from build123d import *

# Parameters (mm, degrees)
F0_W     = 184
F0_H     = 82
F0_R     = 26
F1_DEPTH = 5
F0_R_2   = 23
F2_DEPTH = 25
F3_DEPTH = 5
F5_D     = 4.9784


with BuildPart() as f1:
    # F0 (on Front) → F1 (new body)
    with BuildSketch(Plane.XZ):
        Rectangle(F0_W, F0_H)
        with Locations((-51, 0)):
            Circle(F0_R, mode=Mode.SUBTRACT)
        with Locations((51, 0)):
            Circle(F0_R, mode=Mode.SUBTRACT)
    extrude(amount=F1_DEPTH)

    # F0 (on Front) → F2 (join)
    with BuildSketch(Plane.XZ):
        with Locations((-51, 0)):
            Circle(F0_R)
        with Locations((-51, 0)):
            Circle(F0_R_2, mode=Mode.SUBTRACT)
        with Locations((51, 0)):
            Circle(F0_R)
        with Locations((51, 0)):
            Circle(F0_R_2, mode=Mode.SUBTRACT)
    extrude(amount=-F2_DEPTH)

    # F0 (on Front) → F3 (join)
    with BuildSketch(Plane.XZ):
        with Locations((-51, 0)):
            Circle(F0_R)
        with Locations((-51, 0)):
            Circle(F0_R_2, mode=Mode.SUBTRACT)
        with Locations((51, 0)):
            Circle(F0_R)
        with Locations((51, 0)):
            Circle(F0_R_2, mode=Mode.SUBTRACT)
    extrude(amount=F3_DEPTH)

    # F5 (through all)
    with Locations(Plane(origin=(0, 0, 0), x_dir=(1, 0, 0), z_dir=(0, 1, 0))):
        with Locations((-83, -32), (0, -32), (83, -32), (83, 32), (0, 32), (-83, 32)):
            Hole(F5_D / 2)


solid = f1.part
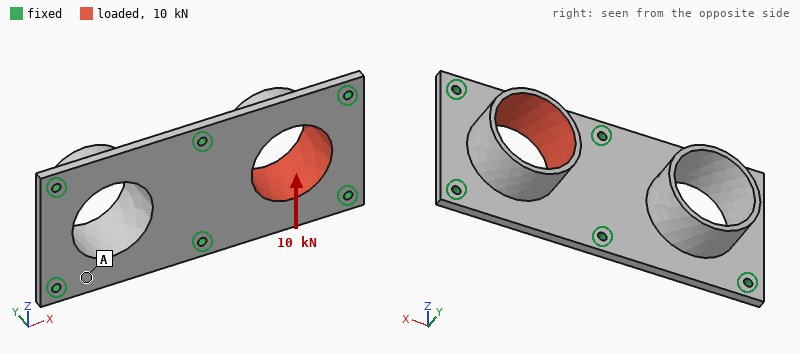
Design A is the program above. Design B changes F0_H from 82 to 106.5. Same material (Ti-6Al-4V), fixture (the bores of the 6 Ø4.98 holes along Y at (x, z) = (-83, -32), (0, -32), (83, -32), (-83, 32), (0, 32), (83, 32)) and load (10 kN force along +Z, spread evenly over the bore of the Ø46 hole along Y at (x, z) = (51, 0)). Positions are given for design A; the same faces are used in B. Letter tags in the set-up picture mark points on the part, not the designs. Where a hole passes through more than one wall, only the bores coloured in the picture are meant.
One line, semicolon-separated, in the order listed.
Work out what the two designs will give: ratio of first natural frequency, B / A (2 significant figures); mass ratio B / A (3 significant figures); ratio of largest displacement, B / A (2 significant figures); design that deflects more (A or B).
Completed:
0.97; 1.28; 0.84; A
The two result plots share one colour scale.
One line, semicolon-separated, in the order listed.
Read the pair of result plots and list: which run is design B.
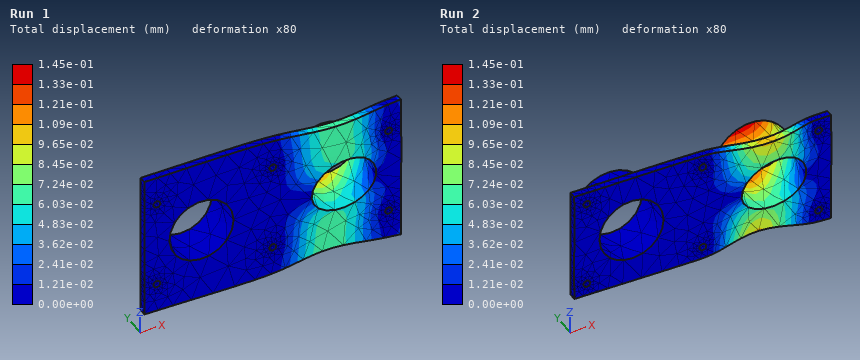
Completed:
Run 1
